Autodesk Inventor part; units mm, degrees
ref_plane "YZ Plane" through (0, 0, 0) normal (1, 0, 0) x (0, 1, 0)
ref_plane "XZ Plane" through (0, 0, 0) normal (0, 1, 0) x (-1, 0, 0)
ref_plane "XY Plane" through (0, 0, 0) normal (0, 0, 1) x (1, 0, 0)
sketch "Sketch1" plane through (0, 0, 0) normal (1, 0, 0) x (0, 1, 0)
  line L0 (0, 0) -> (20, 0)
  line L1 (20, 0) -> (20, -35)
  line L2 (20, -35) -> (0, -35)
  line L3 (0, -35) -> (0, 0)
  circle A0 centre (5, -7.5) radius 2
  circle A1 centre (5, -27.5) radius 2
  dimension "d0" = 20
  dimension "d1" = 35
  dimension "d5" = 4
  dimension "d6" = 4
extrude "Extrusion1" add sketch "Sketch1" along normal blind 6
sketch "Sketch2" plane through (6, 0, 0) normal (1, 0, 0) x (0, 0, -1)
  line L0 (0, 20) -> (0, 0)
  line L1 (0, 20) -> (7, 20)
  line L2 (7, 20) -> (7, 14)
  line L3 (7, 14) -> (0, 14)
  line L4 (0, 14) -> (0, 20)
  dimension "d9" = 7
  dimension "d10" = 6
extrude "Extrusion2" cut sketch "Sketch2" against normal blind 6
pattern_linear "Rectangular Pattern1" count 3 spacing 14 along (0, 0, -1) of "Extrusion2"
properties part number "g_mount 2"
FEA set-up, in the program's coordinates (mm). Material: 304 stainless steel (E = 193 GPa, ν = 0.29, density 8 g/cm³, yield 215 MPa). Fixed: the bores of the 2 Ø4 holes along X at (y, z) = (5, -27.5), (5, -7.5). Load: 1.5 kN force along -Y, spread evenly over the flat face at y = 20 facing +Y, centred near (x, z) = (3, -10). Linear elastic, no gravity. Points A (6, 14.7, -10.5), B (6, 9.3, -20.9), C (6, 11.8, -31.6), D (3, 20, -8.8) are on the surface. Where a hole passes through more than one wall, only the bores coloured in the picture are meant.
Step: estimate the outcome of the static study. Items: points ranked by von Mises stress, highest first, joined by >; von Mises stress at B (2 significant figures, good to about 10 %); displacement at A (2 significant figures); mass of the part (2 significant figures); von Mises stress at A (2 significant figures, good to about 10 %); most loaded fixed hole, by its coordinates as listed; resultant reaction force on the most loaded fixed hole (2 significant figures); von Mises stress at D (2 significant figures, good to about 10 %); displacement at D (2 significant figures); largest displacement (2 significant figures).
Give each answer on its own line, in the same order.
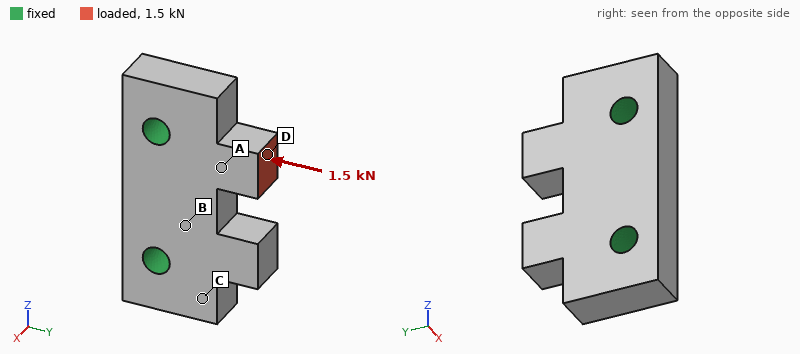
D > A > B > C
7.6 MPa
1.4 µm
26 g
27 MPa
(5, -7.5)
1.3 kN
36 MPa
2.3 µm
2.5 µm
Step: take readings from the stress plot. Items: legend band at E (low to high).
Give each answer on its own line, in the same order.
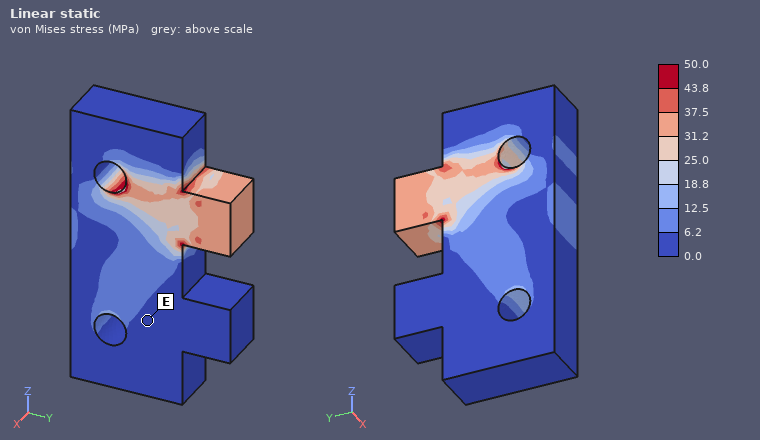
0.0 to 6.2 MPa
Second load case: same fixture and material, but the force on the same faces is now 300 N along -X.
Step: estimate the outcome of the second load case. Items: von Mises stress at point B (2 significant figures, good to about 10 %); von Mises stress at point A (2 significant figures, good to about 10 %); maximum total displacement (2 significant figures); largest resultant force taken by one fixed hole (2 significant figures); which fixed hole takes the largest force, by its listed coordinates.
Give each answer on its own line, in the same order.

12 MPa
35 MPa
8.6 µm
270 N
(5, -7.5)
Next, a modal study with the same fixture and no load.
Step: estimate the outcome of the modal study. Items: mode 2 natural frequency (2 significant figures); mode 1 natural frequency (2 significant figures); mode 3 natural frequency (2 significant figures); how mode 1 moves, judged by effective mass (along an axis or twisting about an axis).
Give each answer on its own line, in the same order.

30 kHz
23 kHz
43 kHz
along X
